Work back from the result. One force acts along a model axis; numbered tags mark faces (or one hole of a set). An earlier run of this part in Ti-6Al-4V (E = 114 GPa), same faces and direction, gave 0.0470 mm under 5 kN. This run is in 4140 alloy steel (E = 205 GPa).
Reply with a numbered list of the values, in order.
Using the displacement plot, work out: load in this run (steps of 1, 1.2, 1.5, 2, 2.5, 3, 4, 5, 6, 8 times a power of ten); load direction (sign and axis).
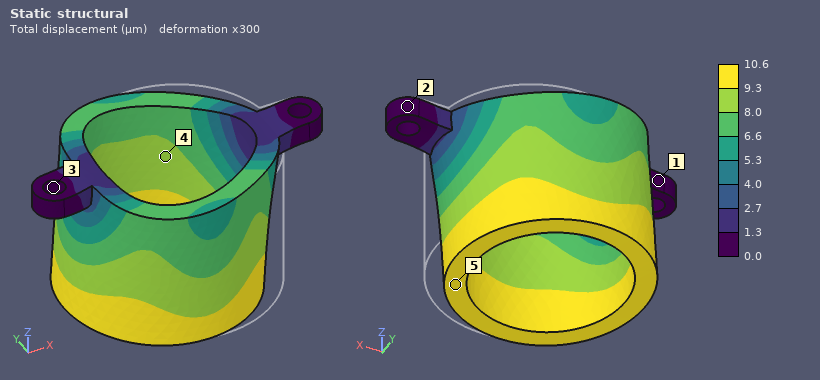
1. 2 kN
2. -X
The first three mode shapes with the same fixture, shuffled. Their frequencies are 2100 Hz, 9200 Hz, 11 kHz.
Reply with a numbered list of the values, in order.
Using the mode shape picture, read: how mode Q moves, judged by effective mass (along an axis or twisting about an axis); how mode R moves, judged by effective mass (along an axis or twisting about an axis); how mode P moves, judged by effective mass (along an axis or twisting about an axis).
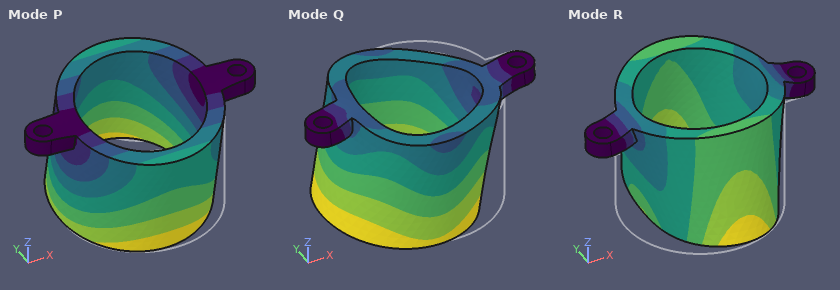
1. along X
2. along Z
3. along Y
